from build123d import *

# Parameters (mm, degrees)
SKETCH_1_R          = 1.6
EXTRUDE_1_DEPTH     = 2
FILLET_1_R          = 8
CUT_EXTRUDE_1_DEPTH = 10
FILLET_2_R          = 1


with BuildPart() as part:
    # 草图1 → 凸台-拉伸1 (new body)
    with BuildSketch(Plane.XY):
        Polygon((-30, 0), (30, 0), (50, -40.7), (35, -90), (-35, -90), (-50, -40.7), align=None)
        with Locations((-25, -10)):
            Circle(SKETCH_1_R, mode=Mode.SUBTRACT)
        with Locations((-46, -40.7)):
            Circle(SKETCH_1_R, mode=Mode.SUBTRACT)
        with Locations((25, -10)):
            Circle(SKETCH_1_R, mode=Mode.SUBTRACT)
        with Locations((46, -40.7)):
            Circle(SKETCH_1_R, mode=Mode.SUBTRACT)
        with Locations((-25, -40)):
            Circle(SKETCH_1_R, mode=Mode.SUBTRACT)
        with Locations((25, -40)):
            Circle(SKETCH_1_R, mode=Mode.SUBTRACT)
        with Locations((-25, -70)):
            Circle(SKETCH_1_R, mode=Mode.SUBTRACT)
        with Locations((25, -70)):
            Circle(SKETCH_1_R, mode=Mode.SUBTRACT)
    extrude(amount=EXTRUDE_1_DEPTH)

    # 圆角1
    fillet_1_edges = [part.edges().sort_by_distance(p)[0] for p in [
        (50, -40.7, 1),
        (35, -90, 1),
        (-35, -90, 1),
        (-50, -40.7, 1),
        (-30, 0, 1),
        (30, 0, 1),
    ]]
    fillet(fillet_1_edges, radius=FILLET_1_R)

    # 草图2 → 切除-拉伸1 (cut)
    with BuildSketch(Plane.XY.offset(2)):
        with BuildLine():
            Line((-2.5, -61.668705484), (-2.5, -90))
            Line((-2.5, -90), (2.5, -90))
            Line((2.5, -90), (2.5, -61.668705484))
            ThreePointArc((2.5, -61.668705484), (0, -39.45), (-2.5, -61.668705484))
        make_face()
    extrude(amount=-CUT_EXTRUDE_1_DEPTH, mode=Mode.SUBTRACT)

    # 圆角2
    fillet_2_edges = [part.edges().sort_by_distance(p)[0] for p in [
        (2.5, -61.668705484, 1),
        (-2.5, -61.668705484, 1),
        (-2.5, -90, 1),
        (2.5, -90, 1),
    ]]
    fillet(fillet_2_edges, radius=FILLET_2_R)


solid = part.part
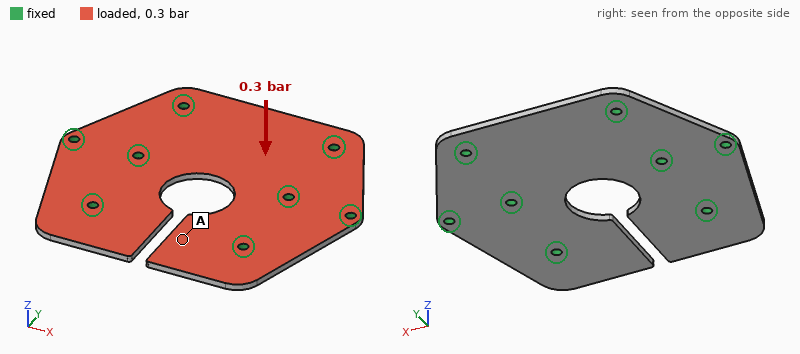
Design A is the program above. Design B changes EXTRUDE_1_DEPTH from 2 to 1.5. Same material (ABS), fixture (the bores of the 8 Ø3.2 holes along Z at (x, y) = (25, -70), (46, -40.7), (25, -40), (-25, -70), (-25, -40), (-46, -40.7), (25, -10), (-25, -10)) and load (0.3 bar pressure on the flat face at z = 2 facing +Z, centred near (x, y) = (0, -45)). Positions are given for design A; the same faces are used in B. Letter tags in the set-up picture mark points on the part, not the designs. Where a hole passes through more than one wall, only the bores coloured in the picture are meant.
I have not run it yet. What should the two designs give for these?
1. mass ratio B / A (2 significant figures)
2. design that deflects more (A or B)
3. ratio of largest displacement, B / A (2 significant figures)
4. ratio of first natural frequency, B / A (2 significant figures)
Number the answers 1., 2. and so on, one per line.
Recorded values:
1. 0.75
2. B
3. 2.3
4. 0.76
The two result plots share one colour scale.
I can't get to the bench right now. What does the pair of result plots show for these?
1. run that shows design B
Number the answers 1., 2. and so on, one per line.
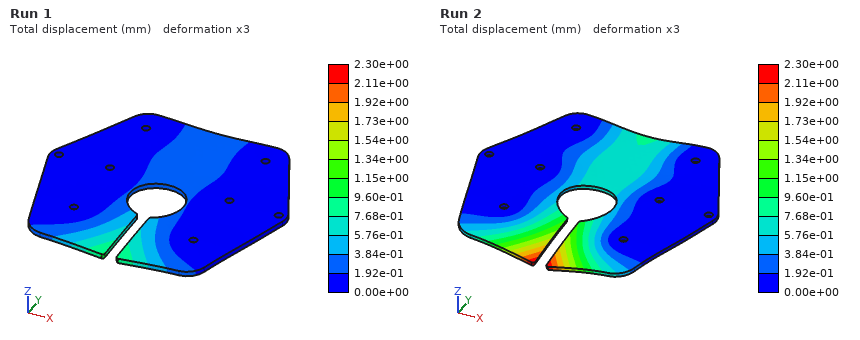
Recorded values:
1. Run 2
